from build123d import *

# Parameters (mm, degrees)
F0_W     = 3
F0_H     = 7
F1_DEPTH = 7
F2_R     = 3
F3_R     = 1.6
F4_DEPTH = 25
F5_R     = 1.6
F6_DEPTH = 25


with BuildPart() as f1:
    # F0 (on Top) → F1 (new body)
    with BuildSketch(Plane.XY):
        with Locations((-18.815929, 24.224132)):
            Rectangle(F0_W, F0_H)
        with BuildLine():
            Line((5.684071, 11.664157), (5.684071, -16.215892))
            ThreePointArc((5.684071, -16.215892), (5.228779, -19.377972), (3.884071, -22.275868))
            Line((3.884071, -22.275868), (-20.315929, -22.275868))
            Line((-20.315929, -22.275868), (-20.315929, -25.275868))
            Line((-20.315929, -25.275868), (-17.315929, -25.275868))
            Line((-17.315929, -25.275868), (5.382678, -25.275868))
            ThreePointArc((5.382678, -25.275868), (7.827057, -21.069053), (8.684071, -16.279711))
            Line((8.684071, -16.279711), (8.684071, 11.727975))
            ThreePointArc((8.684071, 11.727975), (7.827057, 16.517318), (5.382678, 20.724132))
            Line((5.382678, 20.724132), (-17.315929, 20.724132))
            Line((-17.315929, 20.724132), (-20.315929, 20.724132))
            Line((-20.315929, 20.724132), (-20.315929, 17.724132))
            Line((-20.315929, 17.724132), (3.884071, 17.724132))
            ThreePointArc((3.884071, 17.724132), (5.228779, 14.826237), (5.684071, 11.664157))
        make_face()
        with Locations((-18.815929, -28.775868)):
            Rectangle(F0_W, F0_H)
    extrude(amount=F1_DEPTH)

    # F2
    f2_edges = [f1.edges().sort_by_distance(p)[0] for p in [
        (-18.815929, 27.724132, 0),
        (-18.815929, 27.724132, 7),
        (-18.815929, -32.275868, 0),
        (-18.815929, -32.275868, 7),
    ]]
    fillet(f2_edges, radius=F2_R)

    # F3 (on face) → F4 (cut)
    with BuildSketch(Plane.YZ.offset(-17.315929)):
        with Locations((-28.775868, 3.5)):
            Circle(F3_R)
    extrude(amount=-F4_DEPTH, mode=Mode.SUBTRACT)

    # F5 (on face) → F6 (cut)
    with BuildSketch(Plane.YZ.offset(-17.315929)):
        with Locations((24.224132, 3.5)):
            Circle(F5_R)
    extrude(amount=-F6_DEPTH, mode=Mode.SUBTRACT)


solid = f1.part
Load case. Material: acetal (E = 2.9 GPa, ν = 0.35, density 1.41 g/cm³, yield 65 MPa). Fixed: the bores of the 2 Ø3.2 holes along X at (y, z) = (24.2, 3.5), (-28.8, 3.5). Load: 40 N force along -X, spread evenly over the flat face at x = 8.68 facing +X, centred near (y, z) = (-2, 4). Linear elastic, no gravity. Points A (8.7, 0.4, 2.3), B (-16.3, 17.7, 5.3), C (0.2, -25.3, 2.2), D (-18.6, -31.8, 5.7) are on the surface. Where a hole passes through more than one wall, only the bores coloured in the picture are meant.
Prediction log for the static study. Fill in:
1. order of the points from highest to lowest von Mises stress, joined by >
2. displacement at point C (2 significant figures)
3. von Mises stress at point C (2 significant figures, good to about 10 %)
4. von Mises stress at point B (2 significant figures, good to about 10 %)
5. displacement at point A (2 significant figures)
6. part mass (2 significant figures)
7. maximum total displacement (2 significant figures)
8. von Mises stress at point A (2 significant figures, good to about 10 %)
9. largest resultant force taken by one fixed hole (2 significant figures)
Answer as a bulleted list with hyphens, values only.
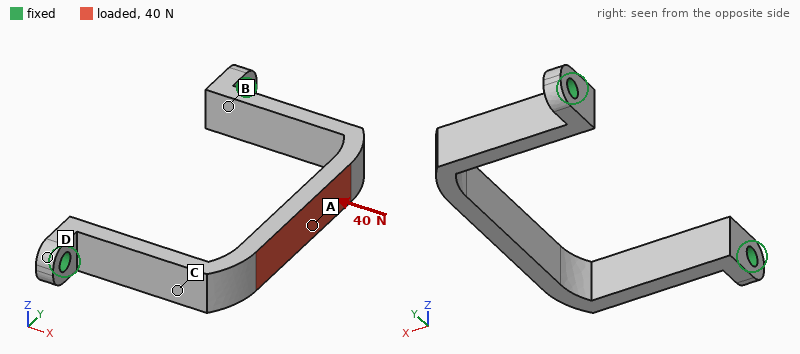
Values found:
- A > C > B > D
- 0.087 mm
- 7.9 MPa
- 3.7 MPa
- 0.41 mm
- 3.1 g
- 0.42 mm
- 12 MPa
- 22 N
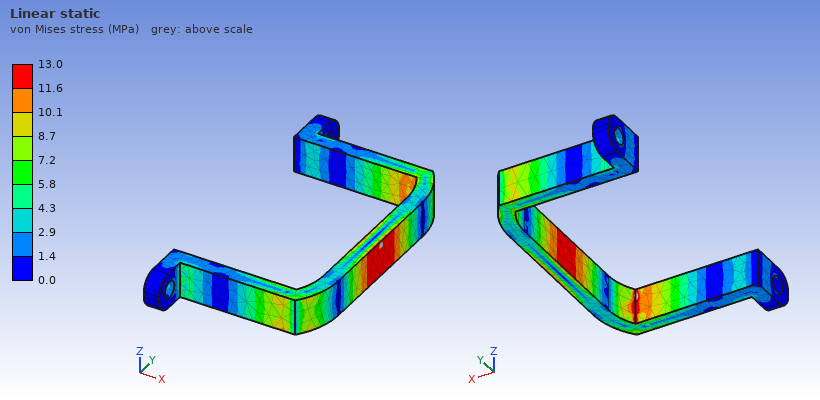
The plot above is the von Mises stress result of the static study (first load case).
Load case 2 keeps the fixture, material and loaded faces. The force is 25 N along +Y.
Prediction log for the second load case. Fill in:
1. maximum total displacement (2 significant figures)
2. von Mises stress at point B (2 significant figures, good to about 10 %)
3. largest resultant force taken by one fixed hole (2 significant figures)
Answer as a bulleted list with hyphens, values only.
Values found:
- 0.72 mm
- 12 MPa
- 15 N
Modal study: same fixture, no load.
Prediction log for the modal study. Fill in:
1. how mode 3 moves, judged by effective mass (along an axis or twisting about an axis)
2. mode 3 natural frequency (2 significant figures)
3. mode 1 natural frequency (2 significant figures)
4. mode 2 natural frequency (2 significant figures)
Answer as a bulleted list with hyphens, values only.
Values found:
- twisting about X
- 1300 Hz
- 720 Hz
- 720 Hz
